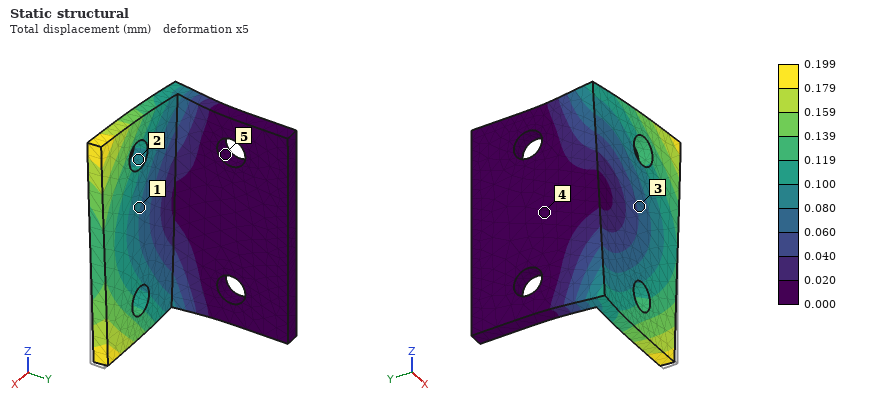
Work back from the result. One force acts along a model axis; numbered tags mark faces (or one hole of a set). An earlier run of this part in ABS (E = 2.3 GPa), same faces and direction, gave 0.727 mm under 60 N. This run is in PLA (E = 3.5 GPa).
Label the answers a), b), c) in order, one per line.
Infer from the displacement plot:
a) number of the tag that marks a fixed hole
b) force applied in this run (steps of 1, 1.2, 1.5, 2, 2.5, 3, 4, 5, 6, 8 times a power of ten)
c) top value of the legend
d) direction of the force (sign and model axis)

a) 5
b) 25 N
c) 0.199 mm
d) +Z
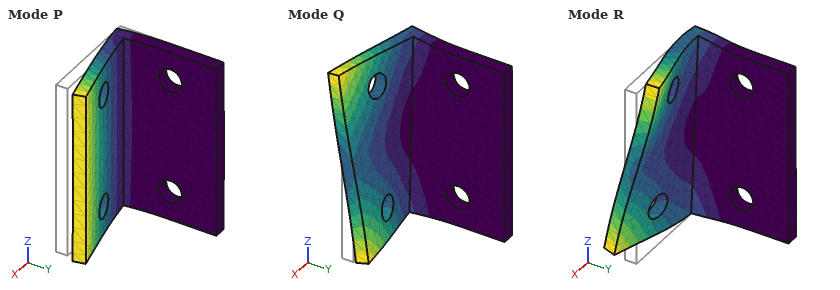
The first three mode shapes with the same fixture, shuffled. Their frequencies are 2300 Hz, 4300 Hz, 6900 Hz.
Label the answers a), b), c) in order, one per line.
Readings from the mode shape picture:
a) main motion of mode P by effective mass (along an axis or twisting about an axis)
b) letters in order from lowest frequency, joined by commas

a) along Y
b) P, Q, R
